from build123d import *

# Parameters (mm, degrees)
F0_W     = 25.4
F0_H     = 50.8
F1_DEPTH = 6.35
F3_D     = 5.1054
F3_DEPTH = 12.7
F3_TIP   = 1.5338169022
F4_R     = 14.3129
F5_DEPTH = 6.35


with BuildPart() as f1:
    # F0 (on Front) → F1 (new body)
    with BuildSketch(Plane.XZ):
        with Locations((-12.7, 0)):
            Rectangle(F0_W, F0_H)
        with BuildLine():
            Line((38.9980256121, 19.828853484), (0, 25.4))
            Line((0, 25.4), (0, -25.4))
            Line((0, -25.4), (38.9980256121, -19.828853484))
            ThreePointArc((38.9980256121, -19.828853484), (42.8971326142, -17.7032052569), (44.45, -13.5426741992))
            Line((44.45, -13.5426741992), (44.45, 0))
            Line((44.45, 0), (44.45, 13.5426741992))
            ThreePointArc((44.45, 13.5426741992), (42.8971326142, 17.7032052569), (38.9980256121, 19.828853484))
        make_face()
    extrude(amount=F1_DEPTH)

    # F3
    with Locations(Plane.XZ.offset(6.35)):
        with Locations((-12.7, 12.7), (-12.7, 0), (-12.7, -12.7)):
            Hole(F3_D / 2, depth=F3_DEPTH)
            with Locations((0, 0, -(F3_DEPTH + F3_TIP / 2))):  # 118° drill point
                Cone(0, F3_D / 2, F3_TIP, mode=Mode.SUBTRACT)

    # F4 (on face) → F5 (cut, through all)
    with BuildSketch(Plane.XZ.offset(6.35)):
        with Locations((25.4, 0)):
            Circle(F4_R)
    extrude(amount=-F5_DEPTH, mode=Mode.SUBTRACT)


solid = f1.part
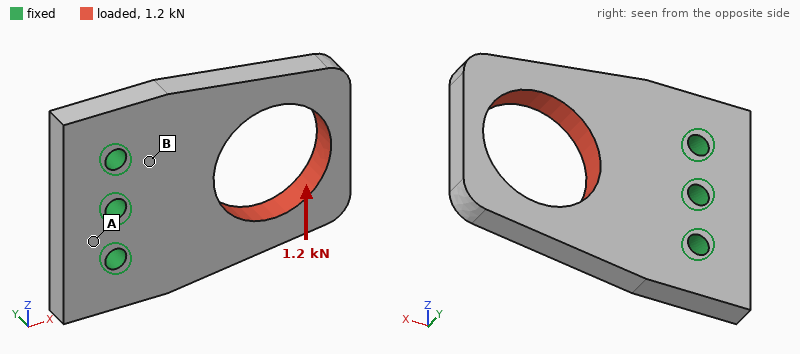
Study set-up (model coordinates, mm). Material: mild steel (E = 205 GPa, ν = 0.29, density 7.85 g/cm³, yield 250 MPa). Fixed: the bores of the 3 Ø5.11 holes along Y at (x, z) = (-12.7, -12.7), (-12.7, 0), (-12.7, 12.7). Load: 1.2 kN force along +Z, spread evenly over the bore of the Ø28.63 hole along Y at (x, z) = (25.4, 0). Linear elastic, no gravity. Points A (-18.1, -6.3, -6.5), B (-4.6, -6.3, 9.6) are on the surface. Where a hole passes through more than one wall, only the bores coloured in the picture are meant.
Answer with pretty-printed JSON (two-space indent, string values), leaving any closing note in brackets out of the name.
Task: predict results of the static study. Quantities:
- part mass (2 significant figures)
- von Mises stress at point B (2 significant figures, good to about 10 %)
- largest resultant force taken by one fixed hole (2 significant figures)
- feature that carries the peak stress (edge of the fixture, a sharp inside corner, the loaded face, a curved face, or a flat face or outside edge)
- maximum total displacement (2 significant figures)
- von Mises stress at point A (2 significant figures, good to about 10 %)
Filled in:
{
  "part mass": "130 g",
  "von Mises stress at point B": "13 MPa",
  "largest resultant force taken by one fixed hole": "1.6 kN",
  "feature that carries the peak stress": "edge of the fixture",
  "maximum total displacement": "16 µm",
  "von Mises stress at point A": "4.8 MPa"
}
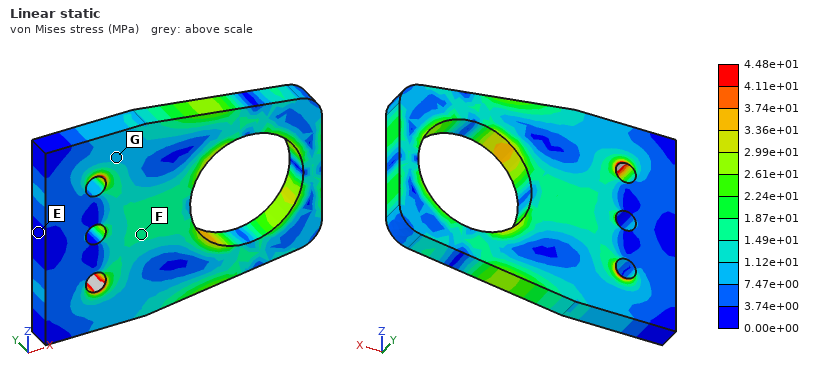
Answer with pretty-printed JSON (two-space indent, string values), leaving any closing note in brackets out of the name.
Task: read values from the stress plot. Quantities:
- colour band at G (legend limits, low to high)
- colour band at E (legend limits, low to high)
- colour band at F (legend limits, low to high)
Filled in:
{
  "colour band at G": "7.47e+00 to 1.12e+01 MPa",
  "colour band at E": "0.00e+00 to 3.74e+00 MPa",
  "colour band at F": "1.49e+01 to 1.87e+01 MPa"
}
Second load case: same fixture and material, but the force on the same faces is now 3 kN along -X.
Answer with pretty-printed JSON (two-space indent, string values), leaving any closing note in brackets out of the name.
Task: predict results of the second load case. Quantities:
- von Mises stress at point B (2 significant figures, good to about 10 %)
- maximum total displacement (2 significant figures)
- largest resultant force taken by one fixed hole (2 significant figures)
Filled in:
{
  "von Mises stress at point B": "9.7 MPa",
  "maximum total displacement": "9.4 µm",
  "largest resultant force taken by one fixed hole": "1.3 kN"
}
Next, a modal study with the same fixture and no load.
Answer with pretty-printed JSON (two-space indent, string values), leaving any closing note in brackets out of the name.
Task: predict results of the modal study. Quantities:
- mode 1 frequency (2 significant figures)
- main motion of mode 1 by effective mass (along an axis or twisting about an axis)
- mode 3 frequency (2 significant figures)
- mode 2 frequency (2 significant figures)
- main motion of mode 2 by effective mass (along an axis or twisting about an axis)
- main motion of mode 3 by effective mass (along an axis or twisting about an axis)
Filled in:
{
  "mode 1 frequency": "2100 Hz",
  "main motion of mode 1 by effective mass": "along Y",
  "mode 3 frequency": "7300 Hz",
  "mode 2 frequency": "4500 Hz",
  "main motion of mode 2 by effective mass": "twisting about X",
  "main motion of mode 3 by effective mass": "along Z"
}
